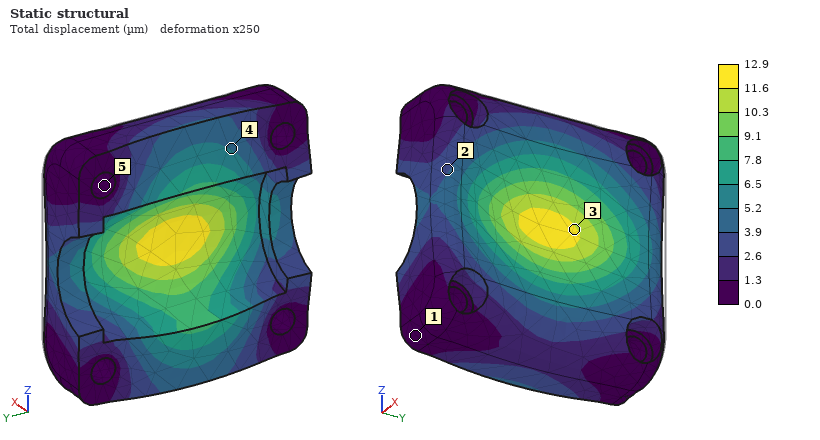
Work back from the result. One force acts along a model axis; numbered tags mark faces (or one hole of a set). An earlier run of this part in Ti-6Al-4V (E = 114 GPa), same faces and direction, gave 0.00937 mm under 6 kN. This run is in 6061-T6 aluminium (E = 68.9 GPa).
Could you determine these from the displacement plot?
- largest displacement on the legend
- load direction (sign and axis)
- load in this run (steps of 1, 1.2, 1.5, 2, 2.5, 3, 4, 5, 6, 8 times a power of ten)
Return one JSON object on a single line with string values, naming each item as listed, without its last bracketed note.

{"largest displacement on the legend": "12.9 µm", "load direction": "-X", "load in this run": "5 kN"}
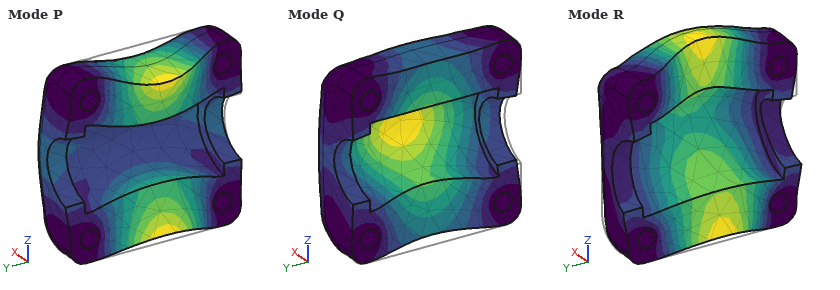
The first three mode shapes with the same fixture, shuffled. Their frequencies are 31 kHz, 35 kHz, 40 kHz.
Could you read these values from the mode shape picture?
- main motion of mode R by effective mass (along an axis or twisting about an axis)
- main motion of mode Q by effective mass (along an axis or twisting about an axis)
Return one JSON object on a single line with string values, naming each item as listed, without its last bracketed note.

{"main motion of mode R by effective mass": "along Z", "main motion of mode Q by effective mass": "along X"}
